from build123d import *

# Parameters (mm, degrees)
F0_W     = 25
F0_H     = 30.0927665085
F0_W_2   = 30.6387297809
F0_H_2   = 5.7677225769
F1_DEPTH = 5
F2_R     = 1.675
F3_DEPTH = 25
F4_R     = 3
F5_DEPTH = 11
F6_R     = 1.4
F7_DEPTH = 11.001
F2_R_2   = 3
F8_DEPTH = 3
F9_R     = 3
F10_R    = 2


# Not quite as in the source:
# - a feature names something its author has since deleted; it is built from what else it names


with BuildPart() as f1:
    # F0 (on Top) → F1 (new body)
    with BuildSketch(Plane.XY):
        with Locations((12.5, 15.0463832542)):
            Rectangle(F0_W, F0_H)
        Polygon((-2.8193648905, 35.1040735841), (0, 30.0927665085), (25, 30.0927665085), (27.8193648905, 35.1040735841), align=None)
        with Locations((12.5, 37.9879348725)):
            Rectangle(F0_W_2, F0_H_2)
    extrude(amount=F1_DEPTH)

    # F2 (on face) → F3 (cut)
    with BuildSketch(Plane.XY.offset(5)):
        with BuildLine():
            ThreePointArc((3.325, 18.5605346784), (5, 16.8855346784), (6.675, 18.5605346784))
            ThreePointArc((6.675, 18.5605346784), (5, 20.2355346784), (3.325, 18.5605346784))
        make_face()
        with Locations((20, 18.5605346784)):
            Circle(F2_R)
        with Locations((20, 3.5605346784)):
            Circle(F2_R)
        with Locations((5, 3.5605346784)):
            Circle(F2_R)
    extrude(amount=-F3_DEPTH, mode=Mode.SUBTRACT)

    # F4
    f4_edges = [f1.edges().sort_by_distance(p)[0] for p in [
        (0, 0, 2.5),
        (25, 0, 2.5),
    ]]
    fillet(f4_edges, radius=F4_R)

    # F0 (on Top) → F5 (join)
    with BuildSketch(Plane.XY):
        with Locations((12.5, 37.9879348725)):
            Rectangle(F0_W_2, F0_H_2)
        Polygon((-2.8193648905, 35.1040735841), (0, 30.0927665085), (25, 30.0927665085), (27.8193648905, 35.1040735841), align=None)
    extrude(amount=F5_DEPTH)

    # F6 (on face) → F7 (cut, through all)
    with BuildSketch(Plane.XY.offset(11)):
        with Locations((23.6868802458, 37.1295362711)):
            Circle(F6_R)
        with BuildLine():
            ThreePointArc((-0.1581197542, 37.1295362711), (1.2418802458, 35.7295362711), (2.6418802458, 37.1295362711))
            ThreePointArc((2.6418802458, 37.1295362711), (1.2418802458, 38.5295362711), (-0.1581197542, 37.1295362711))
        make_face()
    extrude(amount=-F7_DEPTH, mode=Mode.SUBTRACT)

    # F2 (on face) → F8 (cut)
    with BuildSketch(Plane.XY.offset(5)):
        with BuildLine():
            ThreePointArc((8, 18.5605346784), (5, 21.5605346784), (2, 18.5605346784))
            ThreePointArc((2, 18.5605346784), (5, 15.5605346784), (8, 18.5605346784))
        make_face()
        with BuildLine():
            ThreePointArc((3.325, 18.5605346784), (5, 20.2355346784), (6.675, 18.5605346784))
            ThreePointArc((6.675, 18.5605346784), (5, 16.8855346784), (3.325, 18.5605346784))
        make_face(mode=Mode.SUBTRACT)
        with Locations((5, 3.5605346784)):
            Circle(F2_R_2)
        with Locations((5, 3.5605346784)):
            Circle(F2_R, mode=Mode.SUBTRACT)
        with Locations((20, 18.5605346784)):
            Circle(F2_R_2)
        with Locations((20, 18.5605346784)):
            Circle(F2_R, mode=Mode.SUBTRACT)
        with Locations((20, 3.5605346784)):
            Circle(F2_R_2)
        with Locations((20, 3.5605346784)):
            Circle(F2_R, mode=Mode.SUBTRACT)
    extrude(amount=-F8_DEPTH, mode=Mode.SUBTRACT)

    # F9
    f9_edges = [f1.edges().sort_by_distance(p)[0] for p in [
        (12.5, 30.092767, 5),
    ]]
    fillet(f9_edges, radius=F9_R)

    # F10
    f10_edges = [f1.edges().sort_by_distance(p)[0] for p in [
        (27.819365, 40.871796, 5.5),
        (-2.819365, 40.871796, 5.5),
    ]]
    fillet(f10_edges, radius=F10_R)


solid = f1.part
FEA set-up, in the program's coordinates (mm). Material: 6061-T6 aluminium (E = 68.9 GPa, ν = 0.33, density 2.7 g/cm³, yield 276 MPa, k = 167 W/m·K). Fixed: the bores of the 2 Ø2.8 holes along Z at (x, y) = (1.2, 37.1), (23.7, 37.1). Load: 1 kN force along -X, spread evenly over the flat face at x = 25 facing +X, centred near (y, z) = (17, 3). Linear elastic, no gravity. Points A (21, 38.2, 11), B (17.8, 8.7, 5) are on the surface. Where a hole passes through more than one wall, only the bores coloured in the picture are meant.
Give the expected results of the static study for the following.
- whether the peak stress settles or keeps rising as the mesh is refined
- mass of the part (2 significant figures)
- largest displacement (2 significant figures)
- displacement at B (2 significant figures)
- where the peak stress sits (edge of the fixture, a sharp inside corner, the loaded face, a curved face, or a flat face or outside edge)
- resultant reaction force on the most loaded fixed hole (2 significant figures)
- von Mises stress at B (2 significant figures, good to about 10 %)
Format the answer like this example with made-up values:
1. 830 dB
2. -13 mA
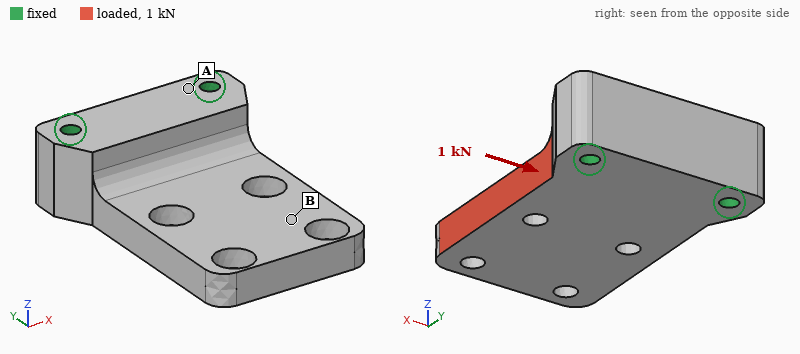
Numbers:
1. keeps rising
2. 18 g
3. 22 µm
4. 16 µm
5. edge of the fixture
6. 1.0 kN
7. 9.8 MPa
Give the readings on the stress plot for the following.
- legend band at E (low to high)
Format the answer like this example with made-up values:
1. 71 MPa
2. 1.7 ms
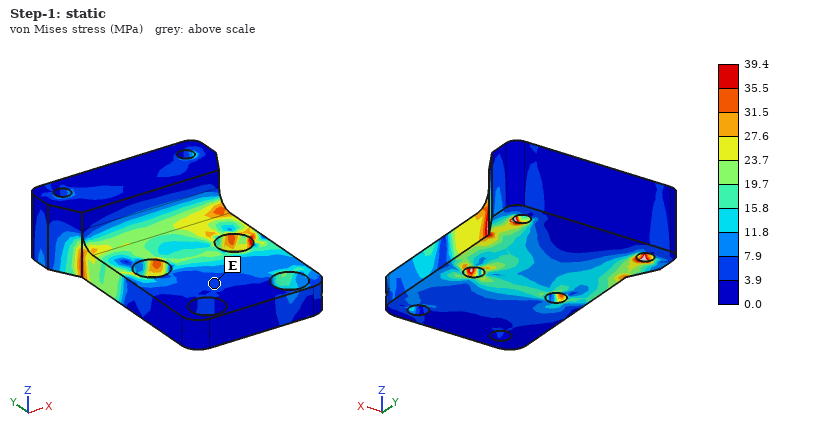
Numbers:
1. 3.9 to 7.9 MPa
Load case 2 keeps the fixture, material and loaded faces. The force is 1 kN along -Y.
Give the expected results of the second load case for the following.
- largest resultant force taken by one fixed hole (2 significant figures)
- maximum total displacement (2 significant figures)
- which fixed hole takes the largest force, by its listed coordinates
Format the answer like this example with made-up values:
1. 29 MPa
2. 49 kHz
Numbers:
1. 1.1 kN
2. 20 µm
3. (23.7, 37.1)
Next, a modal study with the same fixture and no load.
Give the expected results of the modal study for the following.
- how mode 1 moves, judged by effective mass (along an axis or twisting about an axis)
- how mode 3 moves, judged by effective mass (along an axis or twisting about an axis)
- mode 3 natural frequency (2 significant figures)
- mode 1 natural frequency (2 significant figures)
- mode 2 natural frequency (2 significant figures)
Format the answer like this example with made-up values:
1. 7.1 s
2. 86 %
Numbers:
1. along Z
2. along X
3. 14 kHz
4. 4100 Hz
5. 11 kHz
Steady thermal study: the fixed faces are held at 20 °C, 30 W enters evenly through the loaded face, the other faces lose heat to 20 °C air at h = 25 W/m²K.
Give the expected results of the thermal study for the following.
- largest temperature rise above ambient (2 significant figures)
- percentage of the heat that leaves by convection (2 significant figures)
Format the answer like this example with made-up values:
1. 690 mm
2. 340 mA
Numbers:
1. 39 K
2. 3.9 %
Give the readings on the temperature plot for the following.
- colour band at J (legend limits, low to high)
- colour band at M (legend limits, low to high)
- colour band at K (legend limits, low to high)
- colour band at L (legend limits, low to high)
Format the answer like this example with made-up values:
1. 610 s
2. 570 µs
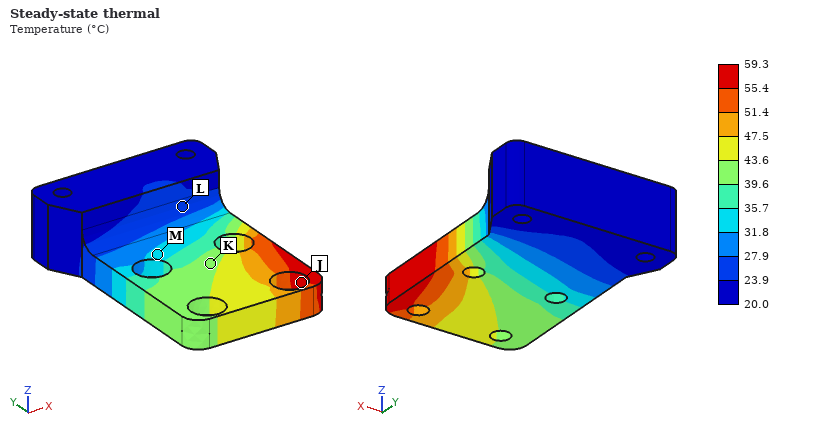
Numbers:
1. 55.4 to 59.3 °C
2. 31.8 to 35.7 °C
3. 39.6 to 43.6 °C
4. 23.9 to 27.9 °C
